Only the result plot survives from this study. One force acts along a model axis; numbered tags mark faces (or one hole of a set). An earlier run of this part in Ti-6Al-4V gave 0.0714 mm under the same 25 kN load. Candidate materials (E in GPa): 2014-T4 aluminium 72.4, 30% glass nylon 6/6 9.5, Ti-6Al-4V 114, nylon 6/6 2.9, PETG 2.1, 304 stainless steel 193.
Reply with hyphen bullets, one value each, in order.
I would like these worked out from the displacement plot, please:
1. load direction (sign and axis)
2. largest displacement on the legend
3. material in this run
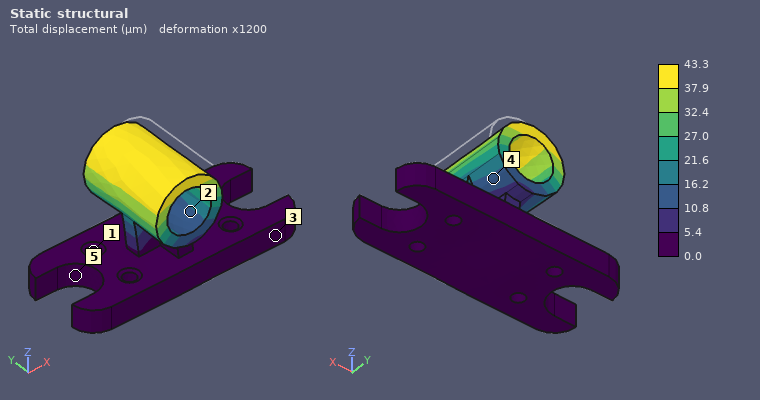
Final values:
- -X
- 43.3 µm
- 304 stainless steel
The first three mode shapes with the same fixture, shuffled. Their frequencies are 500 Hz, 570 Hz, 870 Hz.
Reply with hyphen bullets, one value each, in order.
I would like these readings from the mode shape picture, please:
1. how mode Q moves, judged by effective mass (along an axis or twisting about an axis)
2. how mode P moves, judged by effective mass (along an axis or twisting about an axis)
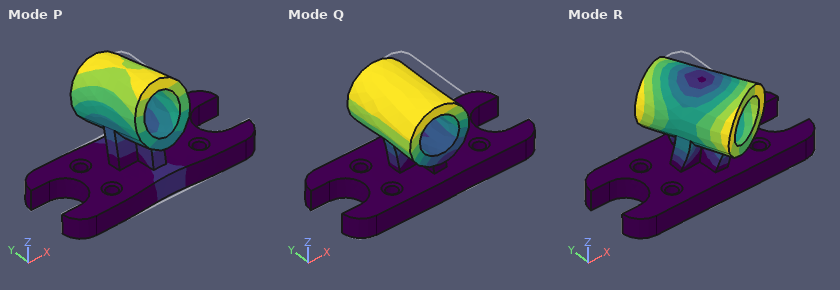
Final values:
- along X
- along Y
